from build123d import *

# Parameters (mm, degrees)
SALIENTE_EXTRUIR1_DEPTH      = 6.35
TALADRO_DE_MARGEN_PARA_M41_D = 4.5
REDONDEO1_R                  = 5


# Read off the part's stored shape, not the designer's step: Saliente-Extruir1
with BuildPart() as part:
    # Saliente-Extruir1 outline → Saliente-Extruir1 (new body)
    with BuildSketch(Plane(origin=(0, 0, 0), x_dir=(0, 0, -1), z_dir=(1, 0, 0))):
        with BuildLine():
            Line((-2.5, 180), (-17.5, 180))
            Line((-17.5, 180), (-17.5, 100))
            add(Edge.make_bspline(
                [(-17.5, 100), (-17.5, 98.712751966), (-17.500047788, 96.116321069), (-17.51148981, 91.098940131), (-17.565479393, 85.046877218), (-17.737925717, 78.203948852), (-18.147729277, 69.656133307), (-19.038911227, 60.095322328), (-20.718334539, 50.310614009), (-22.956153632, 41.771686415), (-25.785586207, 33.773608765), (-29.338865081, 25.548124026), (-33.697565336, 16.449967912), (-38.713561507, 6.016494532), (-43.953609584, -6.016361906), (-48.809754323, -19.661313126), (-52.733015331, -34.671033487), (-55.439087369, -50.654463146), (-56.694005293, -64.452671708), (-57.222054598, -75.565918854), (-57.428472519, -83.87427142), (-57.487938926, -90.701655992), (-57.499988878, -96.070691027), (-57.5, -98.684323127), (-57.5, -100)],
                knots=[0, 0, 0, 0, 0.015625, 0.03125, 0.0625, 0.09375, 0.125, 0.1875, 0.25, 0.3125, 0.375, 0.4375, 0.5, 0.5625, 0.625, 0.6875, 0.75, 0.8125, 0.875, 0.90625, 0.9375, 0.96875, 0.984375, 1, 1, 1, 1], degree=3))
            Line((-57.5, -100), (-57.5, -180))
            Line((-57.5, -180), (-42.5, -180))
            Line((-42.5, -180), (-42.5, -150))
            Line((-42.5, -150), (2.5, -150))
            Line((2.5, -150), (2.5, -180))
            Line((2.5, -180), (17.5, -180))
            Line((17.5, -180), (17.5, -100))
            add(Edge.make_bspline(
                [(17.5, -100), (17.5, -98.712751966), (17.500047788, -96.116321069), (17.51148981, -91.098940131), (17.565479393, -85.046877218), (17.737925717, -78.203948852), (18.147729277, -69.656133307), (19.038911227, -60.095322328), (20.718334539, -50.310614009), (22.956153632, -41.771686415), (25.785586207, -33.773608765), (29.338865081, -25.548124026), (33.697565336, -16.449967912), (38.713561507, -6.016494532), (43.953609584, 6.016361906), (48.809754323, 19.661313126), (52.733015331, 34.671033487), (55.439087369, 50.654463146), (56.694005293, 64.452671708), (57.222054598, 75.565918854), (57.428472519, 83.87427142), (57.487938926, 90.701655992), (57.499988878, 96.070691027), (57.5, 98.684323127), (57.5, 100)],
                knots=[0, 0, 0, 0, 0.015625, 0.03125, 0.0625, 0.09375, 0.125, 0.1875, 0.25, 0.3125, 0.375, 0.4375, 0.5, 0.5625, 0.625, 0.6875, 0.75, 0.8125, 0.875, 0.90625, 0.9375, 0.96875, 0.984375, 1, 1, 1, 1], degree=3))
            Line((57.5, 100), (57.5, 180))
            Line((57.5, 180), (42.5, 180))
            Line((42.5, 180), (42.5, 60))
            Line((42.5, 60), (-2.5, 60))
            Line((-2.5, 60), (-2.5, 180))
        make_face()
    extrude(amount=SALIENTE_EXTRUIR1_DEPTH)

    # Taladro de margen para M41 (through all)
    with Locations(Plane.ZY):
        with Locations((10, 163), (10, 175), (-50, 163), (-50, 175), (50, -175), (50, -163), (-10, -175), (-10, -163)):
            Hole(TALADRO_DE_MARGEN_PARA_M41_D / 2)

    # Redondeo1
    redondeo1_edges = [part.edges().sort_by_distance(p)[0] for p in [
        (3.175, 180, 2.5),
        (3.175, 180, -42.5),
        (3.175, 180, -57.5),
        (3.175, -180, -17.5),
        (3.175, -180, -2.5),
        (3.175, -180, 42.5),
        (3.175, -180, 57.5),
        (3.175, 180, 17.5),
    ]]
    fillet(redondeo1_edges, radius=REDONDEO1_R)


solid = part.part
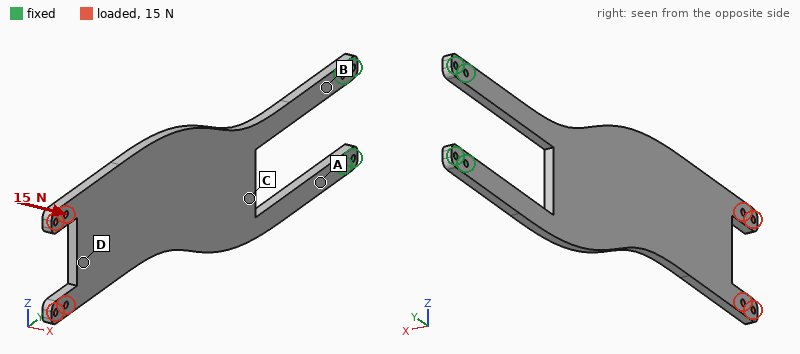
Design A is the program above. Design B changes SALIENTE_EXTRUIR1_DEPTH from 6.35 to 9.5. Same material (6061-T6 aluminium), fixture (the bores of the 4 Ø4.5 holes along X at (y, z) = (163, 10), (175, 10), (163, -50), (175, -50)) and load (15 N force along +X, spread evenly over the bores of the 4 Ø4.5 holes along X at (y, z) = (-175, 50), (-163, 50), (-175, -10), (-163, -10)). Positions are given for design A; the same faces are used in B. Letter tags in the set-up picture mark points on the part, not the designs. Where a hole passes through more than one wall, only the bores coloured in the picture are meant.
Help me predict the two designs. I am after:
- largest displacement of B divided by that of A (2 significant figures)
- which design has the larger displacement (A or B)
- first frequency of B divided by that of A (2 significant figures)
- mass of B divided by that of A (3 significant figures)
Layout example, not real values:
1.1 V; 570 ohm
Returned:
0.30; A; 1.5; 1.50
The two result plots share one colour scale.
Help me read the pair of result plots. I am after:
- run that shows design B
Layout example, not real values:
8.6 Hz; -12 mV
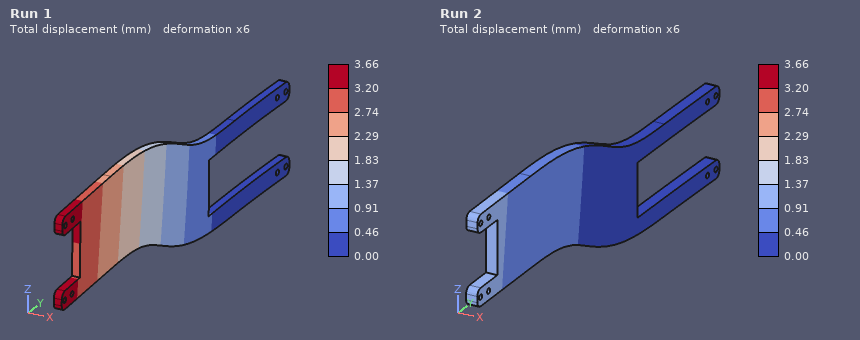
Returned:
Run 2
